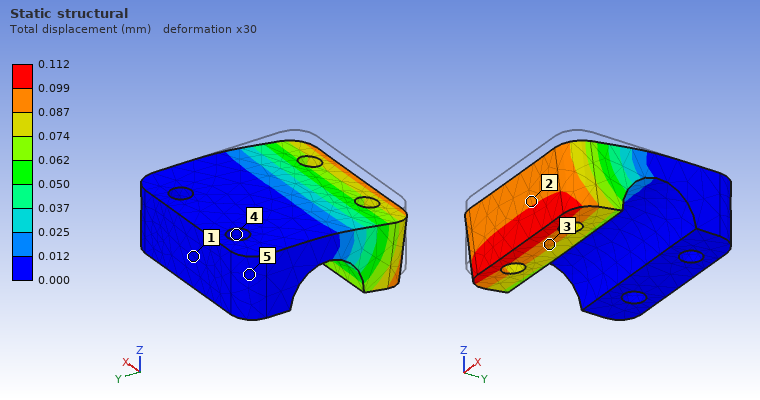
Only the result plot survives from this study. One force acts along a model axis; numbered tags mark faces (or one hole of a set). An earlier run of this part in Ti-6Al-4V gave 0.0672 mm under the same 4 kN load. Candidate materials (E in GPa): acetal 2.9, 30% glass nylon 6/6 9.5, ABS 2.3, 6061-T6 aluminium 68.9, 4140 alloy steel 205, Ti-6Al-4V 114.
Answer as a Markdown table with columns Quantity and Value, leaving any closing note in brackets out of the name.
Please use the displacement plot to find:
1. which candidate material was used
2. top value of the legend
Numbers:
| Quantity | Value |
|---|---|
| which candidate material was used | 6061-T6 aluminium |
| top value of the legend | 0.112 mm |
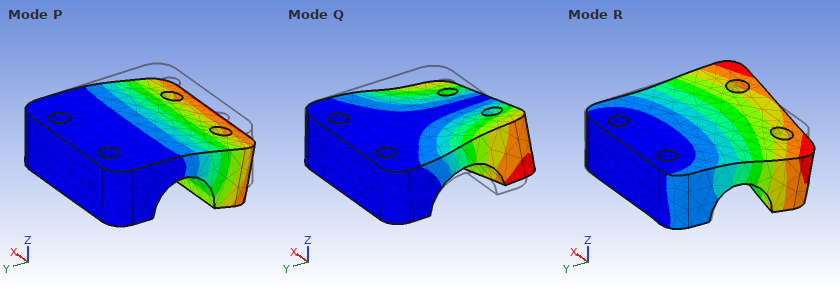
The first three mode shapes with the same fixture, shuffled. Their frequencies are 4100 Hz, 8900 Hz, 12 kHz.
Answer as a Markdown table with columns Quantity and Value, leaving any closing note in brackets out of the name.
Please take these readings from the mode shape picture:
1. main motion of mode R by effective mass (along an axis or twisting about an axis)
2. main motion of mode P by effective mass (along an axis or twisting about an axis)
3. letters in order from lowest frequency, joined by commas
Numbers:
| Quantity | Value |
|---|---|
| main motion of mode R by effective mass | along X |
| main motion of mode P by effective mass | along Z |
| letters in order from lowest frequency, joined by commas | P, Q, R |
